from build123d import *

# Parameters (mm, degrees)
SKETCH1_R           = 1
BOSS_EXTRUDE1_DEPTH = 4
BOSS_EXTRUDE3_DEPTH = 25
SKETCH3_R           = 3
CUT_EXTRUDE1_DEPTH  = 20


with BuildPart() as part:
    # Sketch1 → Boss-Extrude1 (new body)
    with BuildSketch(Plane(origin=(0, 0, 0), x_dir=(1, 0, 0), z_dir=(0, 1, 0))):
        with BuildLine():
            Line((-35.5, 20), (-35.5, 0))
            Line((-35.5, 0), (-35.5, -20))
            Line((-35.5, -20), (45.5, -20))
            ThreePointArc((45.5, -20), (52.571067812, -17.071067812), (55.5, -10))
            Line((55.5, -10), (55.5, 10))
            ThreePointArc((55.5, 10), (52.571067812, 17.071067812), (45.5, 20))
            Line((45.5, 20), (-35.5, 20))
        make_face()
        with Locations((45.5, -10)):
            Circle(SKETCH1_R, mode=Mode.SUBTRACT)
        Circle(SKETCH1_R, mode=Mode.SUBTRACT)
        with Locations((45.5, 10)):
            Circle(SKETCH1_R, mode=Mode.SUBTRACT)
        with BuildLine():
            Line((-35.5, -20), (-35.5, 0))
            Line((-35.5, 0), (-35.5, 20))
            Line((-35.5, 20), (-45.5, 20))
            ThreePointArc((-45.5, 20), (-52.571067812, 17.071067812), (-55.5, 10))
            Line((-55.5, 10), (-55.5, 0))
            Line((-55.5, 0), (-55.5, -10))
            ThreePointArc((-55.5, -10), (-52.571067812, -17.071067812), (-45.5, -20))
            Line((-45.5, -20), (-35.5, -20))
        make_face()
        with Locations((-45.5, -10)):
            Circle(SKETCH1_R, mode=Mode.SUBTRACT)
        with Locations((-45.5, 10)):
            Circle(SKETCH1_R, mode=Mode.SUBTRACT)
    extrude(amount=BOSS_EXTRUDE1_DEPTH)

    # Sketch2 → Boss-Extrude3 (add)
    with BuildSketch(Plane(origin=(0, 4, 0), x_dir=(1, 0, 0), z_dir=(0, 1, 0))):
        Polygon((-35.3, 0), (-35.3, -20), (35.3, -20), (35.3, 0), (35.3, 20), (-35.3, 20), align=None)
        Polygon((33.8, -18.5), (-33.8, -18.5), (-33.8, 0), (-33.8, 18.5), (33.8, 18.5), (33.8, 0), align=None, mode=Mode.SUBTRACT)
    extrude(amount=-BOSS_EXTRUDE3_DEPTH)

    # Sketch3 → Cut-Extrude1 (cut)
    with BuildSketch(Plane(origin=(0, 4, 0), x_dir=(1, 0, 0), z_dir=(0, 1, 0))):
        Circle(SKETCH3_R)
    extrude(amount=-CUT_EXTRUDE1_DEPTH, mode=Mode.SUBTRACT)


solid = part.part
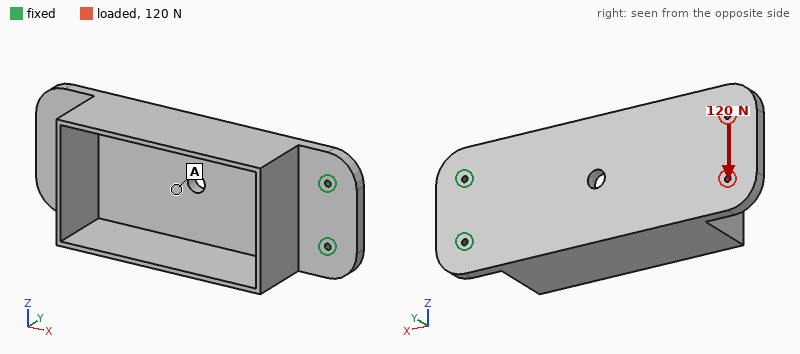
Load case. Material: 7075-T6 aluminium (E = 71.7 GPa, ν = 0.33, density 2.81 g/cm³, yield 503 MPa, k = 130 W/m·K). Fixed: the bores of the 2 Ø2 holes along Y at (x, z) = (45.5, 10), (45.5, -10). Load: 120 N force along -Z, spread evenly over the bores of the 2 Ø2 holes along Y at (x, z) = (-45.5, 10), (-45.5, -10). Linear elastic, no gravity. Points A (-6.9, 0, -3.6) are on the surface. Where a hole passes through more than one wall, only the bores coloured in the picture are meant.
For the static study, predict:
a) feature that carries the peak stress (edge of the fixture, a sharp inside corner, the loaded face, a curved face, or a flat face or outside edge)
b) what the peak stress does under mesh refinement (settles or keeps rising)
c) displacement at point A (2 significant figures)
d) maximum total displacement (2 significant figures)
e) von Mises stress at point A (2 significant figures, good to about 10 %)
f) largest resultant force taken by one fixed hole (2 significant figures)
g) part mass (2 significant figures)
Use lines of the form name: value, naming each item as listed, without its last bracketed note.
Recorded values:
feature that carries the peak stress: edge of the fixture
what the peak stress does under mesh refinement: keeps rising
displacement at point A: 14 µm
maximum total displacement: 34 µm
von Mises stress at point A: 2.4 MPa
largest resultant force taken by one fixed hole: 530 N
part mass: 68 g
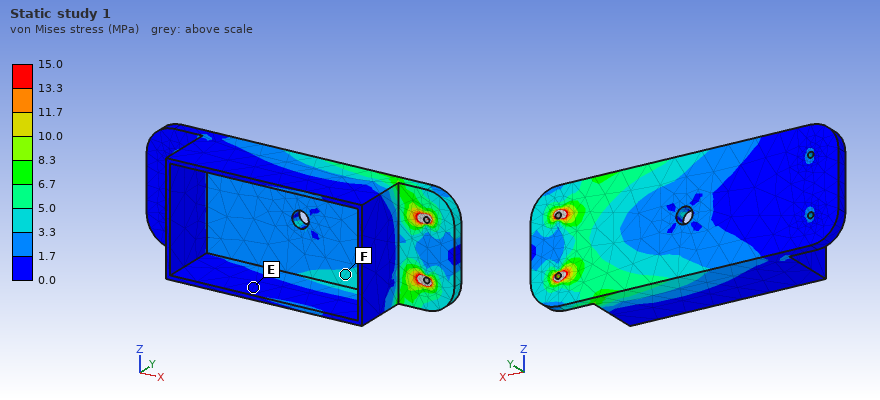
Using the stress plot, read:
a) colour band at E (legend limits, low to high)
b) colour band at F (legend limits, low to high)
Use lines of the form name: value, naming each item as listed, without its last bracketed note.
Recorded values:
colour band at E: 0.0 to 1.7 MPa
colour band at F: 3.3 to 5.0 MPa
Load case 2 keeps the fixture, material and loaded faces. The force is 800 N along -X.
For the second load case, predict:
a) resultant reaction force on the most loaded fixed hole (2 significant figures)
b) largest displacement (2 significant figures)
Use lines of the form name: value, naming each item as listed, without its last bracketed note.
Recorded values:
resultant reaction force on the most loaded fixed hole: 400 N
largest displacement: 18 µm
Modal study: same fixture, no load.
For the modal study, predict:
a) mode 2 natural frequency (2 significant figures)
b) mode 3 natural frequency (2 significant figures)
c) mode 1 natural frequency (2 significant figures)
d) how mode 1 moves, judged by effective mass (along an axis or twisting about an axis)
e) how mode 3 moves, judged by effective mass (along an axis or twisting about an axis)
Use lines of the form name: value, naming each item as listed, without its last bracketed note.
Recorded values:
mode 2 natural frequency: 1200 Hz
mode 3 natural frequency: 2100 Hz
mode 1 natural frequency: 360 Hz
how mode 1 moves, judged by effective mass: along Y
how mode 3 moves, judged by effective mass: along Z
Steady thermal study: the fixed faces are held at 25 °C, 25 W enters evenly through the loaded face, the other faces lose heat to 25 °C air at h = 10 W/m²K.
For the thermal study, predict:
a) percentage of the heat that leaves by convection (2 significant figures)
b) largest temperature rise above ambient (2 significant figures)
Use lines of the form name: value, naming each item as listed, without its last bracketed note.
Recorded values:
percentage of the heat that leaves by convection: 28 %
largest temperature rise above ambient: 82 K
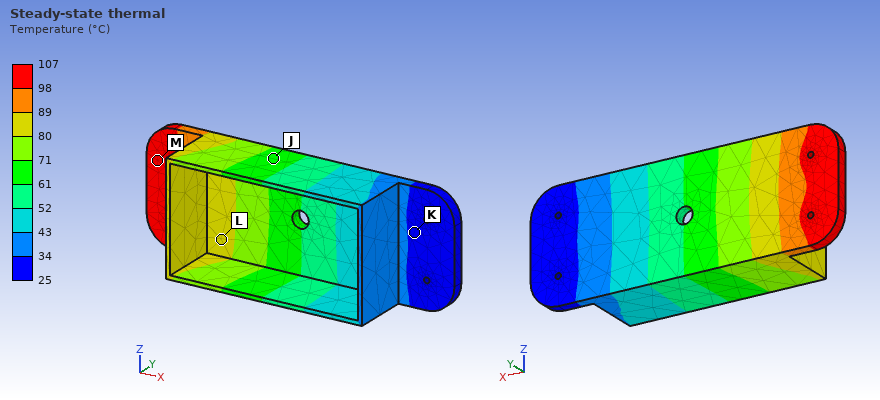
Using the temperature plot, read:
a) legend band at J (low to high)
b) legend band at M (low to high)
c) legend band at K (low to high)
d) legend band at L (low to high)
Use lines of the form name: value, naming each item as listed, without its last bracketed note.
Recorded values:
legend band at J: 61 to 71 °C
legend band at M: 98 to 107 °C
legend band at K: 25 to 34 °C
legend band at L: 80 to 89 °C
